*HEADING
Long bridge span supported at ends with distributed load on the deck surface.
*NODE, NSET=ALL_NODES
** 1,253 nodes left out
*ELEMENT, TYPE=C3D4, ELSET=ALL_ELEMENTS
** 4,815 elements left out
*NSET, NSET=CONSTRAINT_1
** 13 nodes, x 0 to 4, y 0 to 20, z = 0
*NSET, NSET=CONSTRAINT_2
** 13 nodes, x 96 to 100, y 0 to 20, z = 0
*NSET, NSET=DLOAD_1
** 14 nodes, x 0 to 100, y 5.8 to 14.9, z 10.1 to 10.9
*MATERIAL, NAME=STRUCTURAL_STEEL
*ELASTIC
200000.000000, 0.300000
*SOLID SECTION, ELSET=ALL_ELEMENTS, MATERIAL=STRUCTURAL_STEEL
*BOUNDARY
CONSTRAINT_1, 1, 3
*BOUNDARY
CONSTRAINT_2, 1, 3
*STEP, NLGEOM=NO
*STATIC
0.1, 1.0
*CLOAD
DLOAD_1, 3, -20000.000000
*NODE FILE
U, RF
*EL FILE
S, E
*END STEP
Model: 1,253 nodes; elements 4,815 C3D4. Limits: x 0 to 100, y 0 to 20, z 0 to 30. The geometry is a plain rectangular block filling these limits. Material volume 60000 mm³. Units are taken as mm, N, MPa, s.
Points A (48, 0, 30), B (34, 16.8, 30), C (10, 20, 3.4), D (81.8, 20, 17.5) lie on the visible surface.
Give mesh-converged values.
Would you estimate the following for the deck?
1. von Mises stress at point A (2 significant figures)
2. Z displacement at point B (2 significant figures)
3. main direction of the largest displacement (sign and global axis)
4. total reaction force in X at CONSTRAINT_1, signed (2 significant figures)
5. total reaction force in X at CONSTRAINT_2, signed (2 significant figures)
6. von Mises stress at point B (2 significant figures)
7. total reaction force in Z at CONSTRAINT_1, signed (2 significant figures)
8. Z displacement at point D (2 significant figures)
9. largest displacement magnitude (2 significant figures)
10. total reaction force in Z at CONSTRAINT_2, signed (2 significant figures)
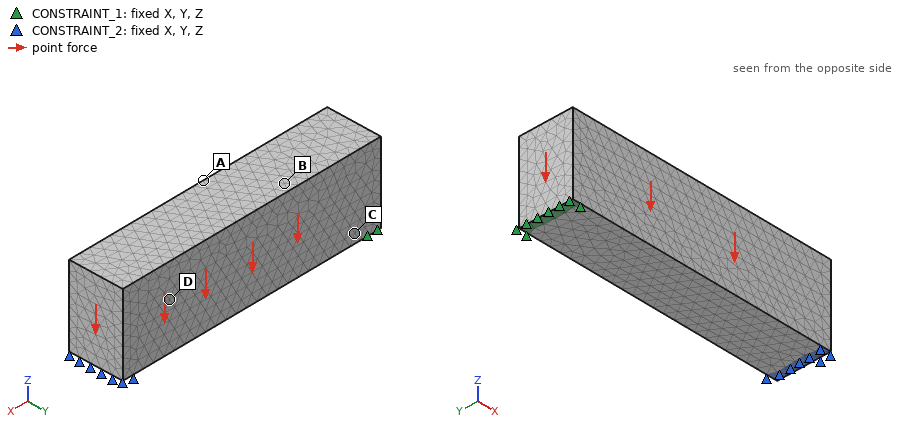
440 MPa
-0.16 mm
-Z
61000 N
-61000 N
360 MPa
1.4e+05 N
-0.13 mm
0.20 mm
1.4e+05 N
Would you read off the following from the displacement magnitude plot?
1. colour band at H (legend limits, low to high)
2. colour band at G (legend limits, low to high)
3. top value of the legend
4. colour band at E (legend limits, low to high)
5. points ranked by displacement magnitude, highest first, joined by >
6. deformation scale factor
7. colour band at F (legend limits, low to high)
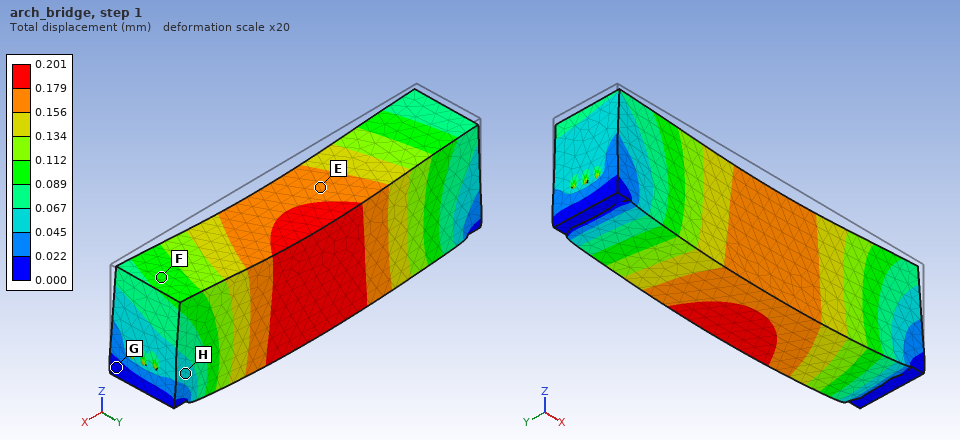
0.045 to 0.067 mm
0.000 to 0.022 mm
0.201 mm
0.156 to 0.179 mm
E > F > H > G
20
0.089 to 0.112 mm
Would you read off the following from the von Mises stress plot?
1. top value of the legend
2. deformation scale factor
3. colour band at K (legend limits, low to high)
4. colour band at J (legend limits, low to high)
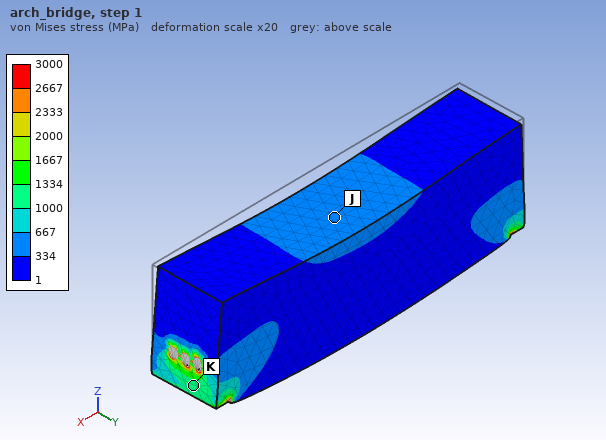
3000 MPa
20
1000 to 1334 MPa
334 to 667 MPa
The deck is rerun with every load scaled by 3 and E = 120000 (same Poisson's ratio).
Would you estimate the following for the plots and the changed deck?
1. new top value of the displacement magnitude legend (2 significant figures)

1.0 mm
